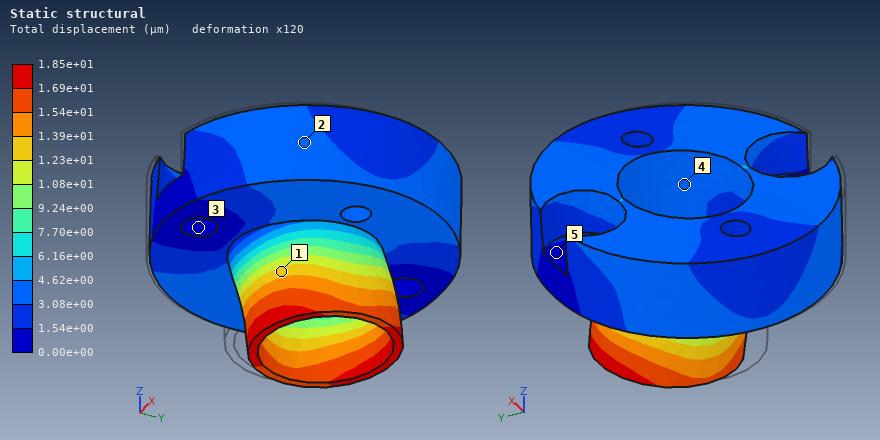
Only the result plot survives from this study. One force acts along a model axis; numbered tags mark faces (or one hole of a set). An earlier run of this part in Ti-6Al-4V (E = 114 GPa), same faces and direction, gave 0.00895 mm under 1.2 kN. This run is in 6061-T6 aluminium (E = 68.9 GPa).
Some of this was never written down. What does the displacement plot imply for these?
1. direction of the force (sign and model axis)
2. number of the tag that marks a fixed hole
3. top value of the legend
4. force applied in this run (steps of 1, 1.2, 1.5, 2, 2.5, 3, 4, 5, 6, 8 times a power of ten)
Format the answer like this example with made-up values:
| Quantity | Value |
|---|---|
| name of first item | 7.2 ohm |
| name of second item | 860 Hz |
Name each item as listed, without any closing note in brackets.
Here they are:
| Quantity | Value |
|---|---|
| direction of the force | +Y |
| number of the tag that marks a fixed hole | 3 |
| top value of the legend | 1.85e+01 µm |
| force applied in this run | 1.5 kN |
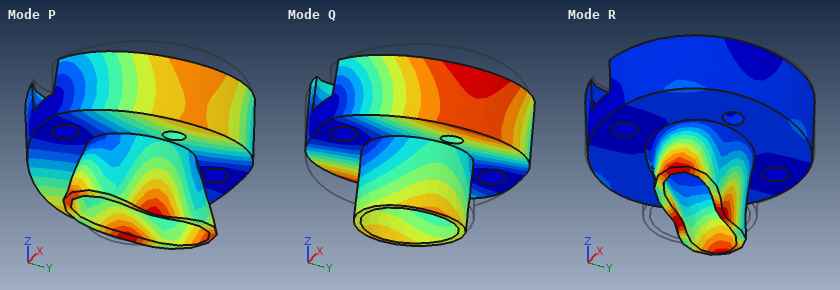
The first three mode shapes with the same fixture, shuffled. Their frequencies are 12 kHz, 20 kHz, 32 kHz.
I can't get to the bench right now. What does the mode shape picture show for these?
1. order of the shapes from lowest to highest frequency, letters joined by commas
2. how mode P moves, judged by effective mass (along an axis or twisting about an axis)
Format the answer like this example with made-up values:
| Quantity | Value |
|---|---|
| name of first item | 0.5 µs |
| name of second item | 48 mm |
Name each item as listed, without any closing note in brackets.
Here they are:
| Quantity | Value |
|---|---|
| order of the shapes from lowest to highest frequency, letters joined by commas | Q, P, R |
| how mode P moves, judged by effective mass | along Z |
